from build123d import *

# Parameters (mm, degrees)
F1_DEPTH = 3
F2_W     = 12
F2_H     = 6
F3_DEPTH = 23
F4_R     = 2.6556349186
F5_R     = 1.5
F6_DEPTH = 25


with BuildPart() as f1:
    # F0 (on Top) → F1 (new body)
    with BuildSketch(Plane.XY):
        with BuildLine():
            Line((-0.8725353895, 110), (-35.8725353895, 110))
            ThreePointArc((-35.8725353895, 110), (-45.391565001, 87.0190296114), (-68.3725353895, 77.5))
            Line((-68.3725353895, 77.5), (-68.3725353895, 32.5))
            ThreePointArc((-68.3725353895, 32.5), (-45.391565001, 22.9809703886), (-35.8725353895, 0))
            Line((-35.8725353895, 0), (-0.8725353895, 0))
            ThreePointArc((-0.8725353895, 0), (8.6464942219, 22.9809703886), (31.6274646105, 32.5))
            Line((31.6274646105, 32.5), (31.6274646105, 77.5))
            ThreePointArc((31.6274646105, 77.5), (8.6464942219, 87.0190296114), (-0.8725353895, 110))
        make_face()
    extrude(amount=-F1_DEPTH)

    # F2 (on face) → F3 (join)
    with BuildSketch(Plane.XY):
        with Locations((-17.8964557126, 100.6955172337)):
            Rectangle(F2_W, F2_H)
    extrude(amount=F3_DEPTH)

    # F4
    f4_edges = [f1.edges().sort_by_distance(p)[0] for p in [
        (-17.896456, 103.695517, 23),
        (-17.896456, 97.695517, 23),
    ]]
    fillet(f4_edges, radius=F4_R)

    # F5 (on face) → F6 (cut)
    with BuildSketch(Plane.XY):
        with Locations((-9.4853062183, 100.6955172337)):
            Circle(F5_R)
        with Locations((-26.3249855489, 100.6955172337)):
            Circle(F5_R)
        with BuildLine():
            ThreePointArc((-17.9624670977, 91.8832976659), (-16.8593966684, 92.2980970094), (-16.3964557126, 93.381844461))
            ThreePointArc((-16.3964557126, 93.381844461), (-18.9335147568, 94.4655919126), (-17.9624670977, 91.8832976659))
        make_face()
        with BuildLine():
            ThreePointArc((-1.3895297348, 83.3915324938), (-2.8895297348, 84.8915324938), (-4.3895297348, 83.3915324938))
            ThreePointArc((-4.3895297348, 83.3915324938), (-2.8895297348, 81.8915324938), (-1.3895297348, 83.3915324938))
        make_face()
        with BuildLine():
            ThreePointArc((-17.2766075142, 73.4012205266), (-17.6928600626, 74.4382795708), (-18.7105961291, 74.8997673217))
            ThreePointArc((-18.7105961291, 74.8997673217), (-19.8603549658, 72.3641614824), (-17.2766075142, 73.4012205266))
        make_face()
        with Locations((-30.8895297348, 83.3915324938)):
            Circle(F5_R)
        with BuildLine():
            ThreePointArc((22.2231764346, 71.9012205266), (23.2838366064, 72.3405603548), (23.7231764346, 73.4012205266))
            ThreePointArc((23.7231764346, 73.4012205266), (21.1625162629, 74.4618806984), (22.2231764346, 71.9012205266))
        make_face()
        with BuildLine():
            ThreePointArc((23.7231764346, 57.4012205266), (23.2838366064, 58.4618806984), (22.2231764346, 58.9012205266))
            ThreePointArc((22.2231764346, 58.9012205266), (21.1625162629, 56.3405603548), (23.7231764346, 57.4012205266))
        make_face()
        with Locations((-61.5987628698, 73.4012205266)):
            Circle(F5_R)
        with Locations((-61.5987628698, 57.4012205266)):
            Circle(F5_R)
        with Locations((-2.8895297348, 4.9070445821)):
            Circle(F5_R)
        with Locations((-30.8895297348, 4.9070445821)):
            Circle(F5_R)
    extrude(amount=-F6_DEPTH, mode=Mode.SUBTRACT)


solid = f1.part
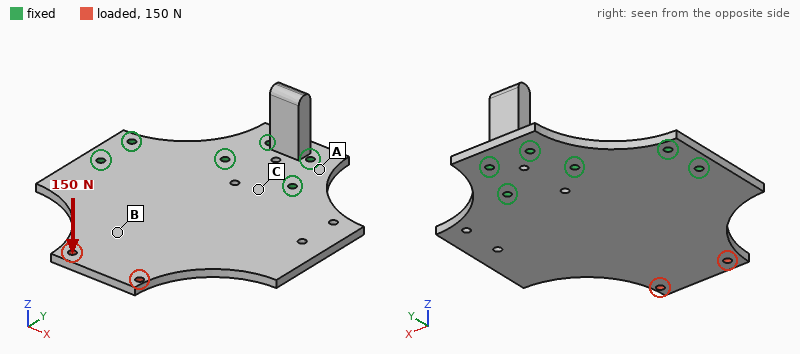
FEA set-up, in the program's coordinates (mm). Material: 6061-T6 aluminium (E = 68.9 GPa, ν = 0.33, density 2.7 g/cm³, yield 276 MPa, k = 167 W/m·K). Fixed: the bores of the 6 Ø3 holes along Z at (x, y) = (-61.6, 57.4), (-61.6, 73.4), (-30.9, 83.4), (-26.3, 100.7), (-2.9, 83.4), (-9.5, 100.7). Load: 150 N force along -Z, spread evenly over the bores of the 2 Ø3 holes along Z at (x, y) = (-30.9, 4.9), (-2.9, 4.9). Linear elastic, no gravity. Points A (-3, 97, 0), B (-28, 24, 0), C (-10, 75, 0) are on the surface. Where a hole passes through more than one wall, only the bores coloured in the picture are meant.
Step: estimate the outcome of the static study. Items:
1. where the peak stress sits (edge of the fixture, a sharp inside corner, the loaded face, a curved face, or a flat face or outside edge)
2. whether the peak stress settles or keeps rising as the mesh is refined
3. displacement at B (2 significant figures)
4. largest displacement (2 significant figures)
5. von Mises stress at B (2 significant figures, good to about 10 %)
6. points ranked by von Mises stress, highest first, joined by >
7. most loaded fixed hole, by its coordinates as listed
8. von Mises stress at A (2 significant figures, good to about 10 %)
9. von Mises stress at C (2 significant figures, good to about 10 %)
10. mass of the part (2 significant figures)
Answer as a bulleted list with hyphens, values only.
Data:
- edge of the fixture
- keeps rising
- 0.73 mm
- 1.6 mm
- 42 MPa
- C > B > A
- (-61.6, 57.4)
- 11 MPa
- 61 MPa
- 66 g
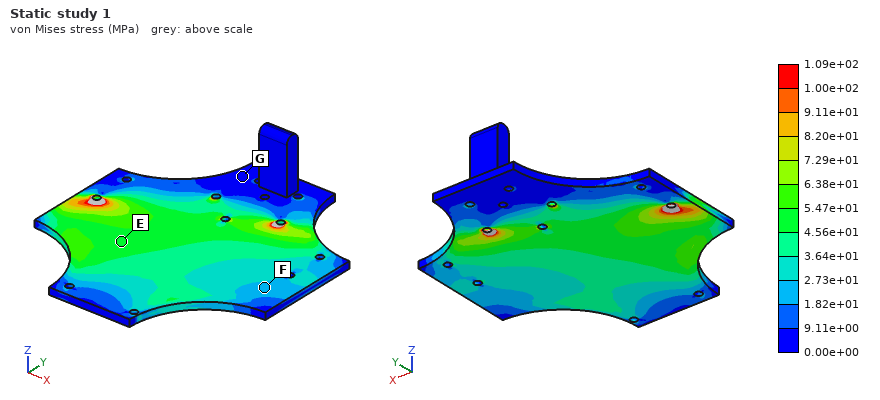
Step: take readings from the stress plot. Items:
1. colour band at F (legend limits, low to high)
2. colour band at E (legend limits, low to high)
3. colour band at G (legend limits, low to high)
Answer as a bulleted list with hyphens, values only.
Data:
- 1.82e+01 to 2.73e+01 MPa
- 4.56e+01 to 5.47e+01 MPa
- 0.00e+00 to 9.11e+00 MPa
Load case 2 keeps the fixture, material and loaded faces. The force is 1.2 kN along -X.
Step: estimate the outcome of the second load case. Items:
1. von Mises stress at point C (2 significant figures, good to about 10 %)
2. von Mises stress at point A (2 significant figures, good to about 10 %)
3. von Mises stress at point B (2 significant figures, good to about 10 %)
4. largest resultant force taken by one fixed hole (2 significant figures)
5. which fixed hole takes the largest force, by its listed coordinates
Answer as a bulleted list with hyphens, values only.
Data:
- 12 MPa
- 9.0 MPa
- 13 MPa
- 1.2 kN
- (-61.6, 57.4)
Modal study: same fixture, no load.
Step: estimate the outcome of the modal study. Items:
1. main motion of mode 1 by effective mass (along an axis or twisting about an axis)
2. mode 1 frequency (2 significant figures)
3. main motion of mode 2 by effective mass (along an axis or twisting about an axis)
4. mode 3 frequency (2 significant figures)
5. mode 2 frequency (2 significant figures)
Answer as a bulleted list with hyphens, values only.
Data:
- along Z
- 550 Hz
- twisting about Y
- 2700 Hz
- 1300 Hz
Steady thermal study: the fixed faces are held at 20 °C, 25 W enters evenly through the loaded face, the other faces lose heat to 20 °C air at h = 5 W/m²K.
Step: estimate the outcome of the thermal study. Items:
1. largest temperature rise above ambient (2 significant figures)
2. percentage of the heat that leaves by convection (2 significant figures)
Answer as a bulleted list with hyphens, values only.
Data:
- 70 K
- 5.5 %
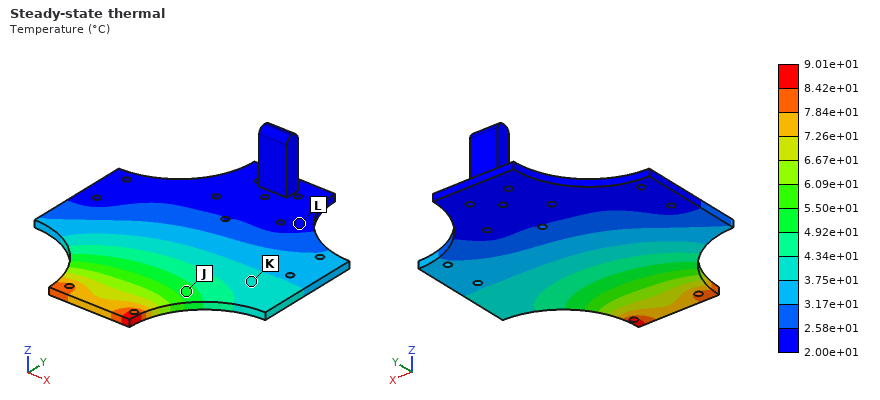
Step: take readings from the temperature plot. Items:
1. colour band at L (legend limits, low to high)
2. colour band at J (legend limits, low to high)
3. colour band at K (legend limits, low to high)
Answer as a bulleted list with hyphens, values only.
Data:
- 2.00e+01 to 2.58e+01 °C
- 4.92e+01 to 5.50e+01 °C
- 3.75e+01 to 4.34e+01 °C
